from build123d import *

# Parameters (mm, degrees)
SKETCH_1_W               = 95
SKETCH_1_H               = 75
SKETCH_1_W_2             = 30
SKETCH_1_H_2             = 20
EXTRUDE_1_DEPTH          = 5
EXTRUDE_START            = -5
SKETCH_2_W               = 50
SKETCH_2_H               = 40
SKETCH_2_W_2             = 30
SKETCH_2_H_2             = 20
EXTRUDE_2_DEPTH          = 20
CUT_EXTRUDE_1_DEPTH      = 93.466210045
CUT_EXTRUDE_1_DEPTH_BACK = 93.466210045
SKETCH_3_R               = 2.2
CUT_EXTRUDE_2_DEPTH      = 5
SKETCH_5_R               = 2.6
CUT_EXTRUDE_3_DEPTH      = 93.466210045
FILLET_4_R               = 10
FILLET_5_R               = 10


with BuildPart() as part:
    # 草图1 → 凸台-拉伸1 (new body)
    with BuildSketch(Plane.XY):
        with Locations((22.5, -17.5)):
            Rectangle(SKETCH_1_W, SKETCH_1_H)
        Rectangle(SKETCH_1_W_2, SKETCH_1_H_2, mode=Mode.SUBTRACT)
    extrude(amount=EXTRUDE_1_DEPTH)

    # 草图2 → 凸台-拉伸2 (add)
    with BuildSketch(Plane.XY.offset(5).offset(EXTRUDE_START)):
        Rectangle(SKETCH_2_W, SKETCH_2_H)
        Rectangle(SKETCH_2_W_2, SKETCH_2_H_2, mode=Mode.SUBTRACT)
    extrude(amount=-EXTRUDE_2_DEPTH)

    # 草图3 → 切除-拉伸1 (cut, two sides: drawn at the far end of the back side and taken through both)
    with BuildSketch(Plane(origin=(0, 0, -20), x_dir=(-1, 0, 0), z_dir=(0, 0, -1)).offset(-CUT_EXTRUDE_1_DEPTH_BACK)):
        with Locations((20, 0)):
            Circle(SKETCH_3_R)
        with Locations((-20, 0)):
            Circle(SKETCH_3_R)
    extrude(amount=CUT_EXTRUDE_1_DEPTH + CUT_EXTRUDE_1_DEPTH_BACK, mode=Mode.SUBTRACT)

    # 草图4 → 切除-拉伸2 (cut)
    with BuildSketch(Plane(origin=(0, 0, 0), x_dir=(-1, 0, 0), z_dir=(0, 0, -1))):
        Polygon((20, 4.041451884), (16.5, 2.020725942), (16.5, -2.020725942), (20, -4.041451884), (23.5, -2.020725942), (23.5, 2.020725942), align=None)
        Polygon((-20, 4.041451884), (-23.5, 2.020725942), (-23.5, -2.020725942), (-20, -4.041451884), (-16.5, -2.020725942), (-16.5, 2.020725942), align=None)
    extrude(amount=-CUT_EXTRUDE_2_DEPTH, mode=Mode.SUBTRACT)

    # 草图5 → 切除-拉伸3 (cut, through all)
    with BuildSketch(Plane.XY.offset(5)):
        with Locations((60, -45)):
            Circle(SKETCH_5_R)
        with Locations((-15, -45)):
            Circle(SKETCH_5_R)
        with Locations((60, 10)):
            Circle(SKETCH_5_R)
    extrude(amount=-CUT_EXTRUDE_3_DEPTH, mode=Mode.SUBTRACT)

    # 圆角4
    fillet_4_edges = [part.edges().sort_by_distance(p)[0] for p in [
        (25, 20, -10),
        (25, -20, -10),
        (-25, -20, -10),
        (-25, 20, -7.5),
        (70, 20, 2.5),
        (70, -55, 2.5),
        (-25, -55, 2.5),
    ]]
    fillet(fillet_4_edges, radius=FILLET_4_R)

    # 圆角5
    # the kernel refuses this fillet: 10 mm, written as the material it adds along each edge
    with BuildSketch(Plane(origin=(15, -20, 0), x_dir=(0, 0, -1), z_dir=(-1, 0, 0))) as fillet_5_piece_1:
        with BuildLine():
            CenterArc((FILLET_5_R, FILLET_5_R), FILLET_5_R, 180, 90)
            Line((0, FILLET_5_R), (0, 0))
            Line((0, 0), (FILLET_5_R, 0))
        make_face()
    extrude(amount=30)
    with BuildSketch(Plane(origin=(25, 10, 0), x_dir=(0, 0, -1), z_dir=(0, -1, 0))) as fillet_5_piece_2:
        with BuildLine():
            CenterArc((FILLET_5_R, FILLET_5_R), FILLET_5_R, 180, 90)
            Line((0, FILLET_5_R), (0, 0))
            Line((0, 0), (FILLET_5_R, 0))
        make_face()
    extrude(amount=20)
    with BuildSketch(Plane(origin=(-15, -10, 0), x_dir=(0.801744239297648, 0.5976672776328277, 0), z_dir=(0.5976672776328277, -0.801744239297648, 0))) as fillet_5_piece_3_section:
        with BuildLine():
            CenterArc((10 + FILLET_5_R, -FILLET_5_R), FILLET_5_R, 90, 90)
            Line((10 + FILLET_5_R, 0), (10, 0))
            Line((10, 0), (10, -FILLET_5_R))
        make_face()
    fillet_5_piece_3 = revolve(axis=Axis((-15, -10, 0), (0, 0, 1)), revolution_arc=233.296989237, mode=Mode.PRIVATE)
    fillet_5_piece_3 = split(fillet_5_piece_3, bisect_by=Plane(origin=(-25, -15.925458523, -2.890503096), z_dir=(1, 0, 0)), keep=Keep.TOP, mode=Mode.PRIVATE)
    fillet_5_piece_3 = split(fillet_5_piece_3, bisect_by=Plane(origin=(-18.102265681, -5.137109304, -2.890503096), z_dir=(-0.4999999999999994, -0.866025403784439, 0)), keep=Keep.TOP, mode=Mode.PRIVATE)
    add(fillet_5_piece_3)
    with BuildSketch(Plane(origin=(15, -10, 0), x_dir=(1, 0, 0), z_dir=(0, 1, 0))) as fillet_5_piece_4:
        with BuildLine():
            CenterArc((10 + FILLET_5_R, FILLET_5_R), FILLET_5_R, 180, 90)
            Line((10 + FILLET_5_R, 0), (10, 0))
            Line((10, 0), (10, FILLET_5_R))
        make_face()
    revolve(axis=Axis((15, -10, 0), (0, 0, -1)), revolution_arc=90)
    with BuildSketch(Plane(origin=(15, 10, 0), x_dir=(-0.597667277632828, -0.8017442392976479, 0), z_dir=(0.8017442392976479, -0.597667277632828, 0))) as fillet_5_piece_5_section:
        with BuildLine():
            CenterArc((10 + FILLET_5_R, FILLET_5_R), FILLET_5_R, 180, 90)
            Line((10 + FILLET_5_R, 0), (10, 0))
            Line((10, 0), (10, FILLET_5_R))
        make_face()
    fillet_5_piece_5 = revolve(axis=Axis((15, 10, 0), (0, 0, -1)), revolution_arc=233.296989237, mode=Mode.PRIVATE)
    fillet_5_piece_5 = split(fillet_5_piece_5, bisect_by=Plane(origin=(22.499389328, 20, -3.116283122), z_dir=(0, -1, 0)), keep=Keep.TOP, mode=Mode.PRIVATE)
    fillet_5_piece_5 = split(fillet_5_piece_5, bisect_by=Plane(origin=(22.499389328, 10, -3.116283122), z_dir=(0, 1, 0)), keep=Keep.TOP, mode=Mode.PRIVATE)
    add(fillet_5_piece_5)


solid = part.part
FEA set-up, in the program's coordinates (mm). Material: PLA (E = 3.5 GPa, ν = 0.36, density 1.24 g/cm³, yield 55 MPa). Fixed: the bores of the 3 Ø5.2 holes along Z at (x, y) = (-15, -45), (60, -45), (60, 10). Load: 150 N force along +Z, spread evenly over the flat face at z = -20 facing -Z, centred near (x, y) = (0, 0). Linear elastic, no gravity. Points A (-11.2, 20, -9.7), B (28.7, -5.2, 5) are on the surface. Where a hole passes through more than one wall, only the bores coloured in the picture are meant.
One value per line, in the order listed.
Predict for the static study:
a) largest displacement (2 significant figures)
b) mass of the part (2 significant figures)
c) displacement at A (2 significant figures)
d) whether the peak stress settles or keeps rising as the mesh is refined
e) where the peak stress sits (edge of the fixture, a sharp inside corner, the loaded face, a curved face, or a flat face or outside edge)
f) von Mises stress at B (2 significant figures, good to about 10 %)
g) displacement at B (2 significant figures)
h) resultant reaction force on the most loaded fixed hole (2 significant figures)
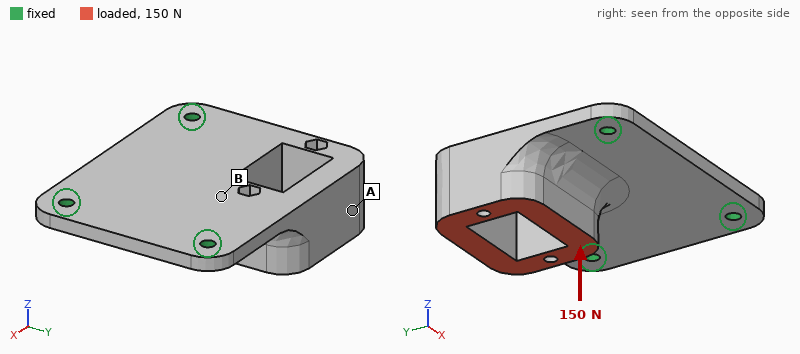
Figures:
0.94 mm
73 g
0.84 mm
keeps rising
edge of the fixture
3.0 MPa
0.21 mm
120 N
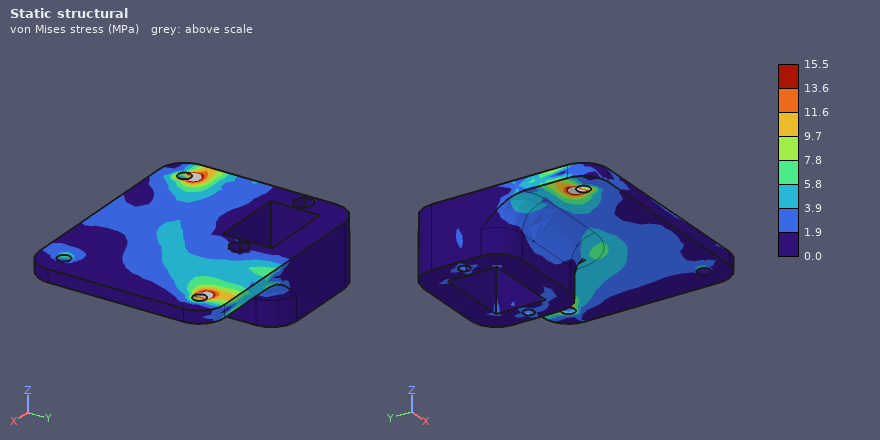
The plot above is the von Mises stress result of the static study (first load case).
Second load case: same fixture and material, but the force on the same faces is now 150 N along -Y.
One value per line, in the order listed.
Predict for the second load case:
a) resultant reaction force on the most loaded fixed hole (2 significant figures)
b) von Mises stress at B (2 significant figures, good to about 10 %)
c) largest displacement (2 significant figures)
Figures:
87 N
1.8 MPa
0.62 mm
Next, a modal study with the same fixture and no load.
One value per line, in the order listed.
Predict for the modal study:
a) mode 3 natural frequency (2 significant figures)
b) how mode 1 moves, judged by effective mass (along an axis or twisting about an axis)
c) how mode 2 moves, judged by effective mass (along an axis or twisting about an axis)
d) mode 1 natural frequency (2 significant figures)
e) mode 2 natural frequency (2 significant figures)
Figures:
1500 Hz
along Z
along Z
380 Hz
1100 Hz
